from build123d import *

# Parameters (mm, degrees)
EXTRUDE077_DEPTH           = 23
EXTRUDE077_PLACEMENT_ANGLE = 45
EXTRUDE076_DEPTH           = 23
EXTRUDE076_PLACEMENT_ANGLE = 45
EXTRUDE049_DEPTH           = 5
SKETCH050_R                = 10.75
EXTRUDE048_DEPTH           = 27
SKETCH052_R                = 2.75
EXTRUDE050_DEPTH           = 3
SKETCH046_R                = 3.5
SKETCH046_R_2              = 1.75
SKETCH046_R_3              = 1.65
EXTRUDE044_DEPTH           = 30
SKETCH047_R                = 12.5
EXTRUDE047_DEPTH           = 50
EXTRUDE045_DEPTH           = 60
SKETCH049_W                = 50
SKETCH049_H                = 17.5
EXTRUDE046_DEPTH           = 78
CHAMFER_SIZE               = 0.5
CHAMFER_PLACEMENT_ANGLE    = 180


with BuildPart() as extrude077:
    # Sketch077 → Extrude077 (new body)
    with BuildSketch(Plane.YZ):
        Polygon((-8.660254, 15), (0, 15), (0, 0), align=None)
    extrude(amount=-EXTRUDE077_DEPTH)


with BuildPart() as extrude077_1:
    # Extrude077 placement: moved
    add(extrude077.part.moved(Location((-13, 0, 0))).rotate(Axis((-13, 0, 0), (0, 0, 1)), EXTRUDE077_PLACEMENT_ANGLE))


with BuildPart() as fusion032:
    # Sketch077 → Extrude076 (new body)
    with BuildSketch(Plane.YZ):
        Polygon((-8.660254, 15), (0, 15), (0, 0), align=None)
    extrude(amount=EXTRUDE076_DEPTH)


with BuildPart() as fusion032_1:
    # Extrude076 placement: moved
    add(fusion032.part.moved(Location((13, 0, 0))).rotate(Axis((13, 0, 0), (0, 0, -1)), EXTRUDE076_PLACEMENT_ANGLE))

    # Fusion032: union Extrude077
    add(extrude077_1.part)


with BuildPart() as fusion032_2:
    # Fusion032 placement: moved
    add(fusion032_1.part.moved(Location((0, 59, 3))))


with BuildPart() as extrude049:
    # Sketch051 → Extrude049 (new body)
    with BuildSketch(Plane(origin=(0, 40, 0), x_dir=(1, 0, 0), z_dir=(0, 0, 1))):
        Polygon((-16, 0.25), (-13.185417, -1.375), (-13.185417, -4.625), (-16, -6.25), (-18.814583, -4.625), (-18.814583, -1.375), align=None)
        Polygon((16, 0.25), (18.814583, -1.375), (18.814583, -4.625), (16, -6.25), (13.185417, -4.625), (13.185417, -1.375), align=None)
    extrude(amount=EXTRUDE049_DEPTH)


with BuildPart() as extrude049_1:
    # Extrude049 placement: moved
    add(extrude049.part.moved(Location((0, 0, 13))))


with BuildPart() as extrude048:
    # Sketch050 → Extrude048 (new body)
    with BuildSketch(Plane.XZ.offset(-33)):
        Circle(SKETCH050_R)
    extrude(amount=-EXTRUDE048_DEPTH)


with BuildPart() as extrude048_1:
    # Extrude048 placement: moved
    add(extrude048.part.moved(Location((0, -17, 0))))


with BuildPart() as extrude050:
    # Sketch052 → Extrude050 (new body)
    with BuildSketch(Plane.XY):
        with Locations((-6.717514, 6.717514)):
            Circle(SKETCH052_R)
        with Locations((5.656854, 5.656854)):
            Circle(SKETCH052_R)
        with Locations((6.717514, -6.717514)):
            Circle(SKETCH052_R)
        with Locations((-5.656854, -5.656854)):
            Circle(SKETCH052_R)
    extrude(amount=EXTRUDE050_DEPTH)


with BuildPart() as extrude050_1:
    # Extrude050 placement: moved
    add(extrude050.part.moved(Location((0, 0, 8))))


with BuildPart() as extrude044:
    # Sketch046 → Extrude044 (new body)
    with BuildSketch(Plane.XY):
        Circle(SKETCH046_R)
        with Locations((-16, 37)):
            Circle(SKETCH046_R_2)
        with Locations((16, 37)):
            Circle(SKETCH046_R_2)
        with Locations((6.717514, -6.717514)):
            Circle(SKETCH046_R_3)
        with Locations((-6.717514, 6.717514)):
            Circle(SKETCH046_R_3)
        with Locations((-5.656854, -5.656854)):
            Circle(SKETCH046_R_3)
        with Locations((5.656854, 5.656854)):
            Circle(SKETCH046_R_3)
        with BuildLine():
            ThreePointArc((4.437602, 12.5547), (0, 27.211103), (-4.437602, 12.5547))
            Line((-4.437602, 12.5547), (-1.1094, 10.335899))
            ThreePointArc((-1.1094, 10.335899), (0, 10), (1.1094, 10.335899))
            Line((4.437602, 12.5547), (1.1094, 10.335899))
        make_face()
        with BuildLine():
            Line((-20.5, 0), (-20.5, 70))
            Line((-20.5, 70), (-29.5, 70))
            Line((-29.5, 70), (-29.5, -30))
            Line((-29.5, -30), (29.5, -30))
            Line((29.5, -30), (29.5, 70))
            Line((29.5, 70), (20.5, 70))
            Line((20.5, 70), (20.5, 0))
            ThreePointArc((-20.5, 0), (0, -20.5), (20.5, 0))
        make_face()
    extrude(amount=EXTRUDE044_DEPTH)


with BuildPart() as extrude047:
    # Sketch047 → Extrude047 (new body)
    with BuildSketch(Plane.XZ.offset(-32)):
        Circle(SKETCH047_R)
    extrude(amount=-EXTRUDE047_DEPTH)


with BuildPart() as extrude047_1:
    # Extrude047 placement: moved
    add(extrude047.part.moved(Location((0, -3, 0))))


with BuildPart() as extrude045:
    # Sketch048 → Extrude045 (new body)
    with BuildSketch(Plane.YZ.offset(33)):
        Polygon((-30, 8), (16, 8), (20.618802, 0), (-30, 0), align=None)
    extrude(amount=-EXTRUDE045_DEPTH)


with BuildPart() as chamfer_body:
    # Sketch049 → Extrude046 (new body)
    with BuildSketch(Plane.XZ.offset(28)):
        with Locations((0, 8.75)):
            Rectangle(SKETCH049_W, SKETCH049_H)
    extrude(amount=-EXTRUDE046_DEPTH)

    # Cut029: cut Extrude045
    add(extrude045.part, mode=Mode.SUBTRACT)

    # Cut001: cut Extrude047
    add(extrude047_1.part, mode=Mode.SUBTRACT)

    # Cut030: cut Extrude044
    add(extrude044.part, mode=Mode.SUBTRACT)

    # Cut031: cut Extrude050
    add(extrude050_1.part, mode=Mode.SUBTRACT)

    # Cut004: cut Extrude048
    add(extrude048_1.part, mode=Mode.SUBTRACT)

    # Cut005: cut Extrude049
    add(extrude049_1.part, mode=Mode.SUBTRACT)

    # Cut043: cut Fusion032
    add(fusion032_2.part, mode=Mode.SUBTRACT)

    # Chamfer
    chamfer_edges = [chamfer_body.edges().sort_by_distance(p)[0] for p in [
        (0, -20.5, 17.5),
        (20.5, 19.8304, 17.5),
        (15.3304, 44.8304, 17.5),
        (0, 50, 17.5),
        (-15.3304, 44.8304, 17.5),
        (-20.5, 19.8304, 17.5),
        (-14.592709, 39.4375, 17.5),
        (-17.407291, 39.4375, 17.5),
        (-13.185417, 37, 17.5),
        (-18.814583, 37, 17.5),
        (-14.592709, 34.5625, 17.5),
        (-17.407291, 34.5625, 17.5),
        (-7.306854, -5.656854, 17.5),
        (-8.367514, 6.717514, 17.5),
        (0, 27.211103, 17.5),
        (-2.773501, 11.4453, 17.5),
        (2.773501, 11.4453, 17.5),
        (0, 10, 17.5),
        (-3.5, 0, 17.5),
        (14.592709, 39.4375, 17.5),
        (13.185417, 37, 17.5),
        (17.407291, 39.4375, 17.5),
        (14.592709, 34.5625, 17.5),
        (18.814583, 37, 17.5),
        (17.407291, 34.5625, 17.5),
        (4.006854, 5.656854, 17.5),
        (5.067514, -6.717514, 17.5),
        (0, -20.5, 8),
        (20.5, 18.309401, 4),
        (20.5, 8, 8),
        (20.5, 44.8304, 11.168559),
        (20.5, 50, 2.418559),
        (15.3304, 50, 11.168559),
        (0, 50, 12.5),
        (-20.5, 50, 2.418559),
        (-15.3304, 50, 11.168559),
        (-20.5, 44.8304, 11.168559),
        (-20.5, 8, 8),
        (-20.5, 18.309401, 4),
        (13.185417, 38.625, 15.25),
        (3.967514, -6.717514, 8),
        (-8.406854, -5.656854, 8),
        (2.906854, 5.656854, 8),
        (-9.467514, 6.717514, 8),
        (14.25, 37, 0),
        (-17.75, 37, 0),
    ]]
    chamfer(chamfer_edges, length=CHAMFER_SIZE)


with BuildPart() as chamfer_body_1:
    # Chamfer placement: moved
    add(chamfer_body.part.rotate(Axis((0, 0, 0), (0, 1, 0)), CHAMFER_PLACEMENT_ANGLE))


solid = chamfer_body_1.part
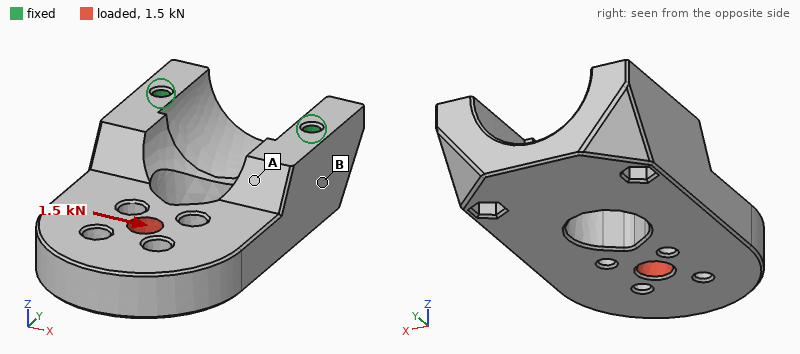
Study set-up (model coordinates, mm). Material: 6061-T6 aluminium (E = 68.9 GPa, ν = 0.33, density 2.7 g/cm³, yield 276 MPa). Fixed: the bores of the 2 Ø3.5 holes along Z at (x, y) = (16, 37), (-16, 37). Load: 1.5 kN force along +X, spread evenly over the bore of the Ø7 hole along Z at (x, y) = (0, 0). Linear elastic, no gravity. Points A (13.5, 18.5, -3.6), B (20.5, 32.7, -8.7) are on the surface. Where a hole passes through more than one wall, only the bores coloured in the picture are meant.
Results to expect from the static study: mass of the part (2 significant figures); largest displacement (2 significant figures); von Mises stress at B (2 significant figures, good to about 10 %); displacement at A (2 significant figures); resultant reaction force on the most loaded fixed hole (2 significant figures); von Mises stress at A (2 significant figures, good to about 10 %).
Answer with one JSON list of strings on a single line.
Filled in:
["69 g", "30 µm", "20 MPa", "11 µm", "1.7 kN", "8.1 MPa"]
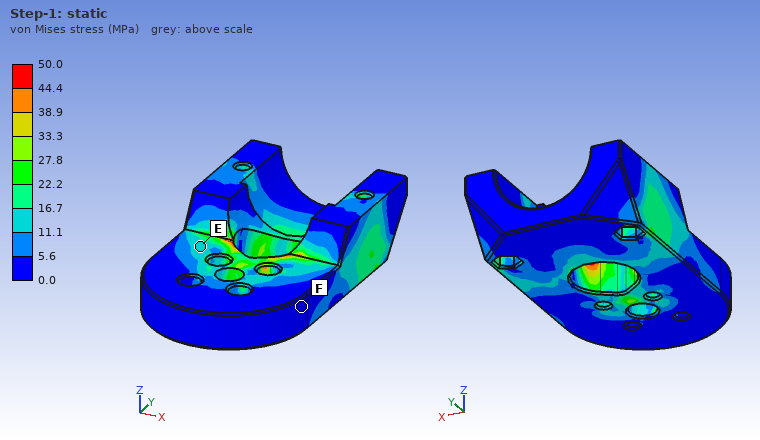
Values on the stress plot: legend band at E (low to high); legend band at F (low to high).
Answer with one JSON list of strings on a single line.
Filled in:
["11.1 to 16.7 MPa", "0.0 to 5.6 MPa"]
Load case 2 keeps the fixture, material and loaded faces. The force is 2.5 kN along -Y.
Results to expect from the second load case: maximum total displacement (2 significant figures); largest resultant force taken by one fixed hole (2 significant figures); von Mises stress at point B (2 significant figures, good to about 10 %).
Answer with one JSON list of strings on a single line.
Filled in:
["19 µm", "1.3 kN", "8.3 MPa"]
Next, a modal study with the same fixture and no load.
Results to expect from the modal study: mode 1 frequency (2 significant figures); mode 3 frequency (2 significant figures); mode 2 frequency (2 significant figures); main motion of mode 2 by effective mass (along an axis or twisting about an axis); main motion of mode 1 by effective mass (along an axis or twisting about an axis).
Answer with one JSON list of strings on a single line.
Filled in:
["3200 Hz", "9200 Hz", "6700 Hz", "along X", "along Z"]
